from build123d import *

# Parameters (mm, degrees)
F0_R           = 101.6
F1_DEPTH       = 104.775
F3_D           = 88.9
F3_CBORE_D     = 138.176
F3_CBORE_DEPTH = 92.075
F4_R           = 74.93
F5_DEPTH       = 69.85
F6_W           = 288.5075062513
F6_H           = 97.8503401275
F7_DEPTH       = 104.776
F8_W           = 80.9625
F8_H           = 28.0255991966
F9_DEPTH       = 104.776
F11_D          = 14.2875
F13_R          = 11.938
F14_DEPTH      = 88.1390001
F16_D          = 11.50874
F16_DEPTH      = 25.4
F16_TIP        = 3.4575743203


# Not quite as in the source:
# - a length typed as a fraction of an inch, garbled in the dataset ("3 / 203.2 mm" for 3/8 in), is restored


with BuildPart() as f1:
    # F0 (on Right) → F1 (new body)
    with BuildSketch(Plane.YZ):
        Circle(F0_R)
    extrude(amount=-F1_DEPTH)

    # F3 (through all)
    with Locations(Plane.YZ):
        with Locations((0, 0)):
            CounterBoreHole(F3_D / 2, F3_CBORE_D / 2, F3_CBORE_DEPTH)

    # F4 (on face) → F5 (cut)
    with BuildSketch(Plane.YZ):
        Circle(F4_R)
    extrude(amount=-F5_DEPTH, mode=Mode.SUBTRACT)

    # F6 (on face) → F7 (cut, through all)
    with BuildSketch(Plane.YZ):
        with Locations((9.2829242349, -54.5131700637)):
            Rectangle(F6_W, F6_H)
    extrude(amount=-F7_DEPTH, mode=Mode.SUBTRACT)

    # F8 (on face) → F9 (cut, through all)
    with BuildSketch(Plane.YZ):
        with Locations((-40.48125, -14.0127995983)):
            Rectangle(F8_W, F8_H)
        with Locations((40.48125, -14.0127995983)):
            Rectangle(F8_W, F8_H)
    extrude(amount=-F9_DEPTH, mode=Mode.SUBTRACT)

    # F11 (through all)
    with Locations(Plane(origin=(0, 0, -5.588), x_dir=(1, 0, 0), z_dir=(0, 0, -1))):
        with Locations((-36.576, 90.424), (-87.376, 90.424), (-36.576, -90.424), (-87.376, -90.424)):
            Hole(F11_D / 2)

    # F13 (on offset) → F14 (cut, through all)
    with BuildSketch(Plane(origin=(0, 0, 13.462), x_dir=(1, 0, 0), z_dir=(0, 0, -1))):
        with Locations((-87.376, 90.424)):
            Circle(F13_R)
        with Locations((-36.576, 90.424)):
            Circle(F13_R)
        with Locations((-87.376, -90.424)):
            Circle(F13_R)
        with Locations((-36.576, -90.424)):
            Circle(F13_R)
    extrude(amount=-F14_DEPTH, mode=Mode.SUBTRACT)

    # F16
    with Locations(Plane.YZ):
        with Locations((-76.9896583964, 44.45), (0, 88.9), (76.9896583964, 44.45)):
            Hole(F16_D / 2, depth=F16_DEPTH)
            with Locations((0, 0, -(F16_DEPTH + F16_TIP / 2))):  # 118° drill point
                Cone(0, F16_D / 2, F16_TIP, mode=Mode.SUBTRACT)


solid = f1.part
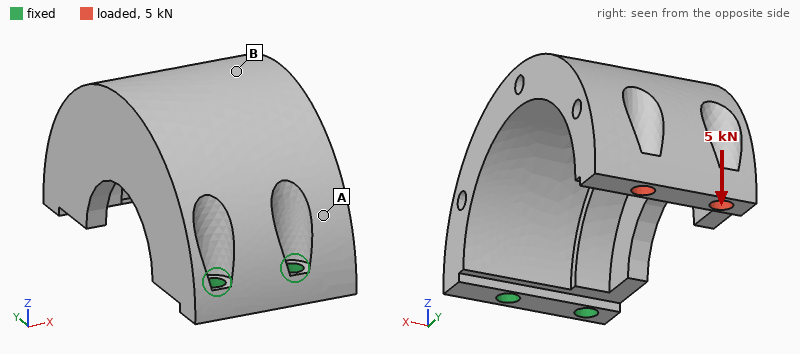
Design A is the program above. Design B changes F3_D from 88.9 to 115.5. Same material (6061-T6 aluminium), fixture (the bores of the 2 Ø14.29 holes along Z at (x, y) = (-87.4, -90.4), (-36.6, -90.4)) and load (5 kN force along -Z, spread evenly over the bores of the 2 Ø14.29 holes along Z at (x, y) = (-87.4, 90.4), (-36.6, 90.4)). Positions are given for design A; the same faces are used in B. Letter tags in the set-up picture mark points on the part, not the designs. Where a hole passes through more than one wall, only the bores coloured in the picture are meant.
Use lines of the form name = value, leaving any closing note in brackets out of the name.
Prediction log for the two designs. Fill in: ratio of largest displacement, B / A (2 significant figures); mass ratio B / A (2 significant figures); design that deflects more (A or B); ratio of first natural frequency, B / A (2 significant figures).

ratio of largest displacement, B / A = 1.2
mass ratio B / A = 0.97
design that deflects more = B
ratio of first natural frequency, B / A = 0.96
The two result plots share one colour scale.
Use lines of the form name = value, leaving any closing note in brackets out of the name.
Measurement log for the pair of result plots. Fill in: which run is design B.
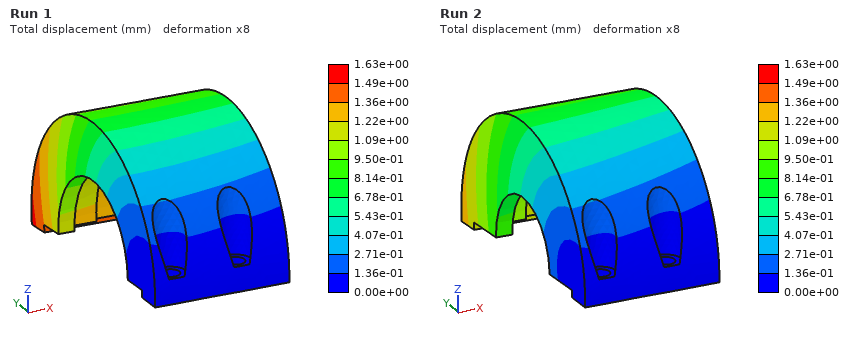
which run is design B = Run 1
